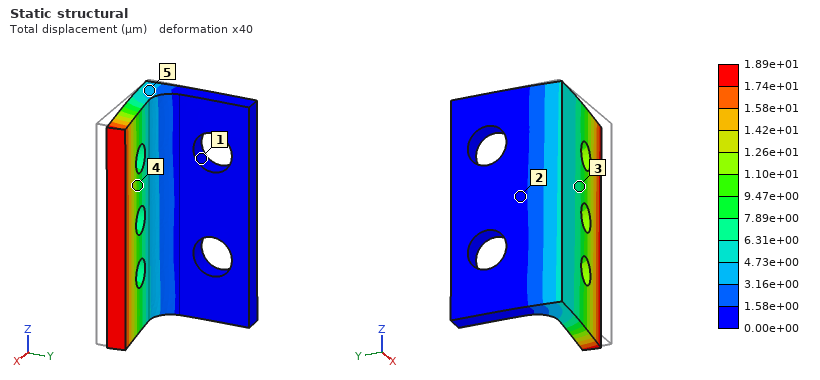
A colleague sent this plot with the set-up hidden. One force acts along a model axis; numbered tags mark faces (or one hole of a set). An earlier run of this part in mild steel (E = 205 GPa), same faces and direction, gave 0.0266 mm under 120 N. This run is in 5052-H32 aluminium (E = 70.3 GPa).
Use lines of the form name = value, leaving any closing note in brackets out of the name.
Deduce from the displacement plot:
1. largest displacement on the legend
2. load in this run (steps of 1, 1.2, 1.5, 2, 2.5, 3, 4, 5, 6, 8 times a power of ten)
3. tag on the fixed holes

largest displacement on the legend = 1.89e+01 µm
load in this run = 30 N
tag on the fixed holes = 1
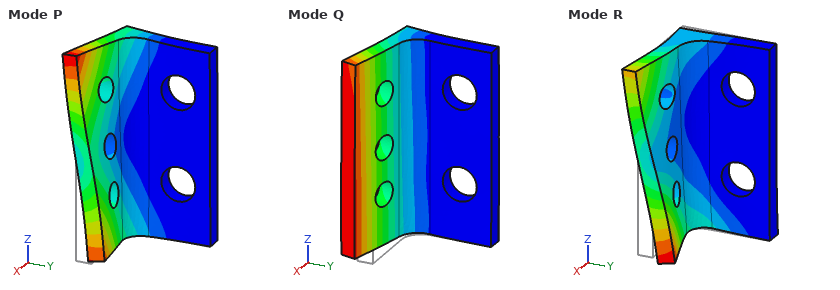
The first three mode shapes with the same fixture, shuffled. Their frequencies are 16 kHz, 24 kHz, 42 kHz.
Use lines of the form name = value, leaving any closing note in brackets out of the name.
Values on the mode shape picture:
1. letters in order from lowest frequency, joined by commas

letters in order from lowest frequency, joined by commas = Q, P, R
